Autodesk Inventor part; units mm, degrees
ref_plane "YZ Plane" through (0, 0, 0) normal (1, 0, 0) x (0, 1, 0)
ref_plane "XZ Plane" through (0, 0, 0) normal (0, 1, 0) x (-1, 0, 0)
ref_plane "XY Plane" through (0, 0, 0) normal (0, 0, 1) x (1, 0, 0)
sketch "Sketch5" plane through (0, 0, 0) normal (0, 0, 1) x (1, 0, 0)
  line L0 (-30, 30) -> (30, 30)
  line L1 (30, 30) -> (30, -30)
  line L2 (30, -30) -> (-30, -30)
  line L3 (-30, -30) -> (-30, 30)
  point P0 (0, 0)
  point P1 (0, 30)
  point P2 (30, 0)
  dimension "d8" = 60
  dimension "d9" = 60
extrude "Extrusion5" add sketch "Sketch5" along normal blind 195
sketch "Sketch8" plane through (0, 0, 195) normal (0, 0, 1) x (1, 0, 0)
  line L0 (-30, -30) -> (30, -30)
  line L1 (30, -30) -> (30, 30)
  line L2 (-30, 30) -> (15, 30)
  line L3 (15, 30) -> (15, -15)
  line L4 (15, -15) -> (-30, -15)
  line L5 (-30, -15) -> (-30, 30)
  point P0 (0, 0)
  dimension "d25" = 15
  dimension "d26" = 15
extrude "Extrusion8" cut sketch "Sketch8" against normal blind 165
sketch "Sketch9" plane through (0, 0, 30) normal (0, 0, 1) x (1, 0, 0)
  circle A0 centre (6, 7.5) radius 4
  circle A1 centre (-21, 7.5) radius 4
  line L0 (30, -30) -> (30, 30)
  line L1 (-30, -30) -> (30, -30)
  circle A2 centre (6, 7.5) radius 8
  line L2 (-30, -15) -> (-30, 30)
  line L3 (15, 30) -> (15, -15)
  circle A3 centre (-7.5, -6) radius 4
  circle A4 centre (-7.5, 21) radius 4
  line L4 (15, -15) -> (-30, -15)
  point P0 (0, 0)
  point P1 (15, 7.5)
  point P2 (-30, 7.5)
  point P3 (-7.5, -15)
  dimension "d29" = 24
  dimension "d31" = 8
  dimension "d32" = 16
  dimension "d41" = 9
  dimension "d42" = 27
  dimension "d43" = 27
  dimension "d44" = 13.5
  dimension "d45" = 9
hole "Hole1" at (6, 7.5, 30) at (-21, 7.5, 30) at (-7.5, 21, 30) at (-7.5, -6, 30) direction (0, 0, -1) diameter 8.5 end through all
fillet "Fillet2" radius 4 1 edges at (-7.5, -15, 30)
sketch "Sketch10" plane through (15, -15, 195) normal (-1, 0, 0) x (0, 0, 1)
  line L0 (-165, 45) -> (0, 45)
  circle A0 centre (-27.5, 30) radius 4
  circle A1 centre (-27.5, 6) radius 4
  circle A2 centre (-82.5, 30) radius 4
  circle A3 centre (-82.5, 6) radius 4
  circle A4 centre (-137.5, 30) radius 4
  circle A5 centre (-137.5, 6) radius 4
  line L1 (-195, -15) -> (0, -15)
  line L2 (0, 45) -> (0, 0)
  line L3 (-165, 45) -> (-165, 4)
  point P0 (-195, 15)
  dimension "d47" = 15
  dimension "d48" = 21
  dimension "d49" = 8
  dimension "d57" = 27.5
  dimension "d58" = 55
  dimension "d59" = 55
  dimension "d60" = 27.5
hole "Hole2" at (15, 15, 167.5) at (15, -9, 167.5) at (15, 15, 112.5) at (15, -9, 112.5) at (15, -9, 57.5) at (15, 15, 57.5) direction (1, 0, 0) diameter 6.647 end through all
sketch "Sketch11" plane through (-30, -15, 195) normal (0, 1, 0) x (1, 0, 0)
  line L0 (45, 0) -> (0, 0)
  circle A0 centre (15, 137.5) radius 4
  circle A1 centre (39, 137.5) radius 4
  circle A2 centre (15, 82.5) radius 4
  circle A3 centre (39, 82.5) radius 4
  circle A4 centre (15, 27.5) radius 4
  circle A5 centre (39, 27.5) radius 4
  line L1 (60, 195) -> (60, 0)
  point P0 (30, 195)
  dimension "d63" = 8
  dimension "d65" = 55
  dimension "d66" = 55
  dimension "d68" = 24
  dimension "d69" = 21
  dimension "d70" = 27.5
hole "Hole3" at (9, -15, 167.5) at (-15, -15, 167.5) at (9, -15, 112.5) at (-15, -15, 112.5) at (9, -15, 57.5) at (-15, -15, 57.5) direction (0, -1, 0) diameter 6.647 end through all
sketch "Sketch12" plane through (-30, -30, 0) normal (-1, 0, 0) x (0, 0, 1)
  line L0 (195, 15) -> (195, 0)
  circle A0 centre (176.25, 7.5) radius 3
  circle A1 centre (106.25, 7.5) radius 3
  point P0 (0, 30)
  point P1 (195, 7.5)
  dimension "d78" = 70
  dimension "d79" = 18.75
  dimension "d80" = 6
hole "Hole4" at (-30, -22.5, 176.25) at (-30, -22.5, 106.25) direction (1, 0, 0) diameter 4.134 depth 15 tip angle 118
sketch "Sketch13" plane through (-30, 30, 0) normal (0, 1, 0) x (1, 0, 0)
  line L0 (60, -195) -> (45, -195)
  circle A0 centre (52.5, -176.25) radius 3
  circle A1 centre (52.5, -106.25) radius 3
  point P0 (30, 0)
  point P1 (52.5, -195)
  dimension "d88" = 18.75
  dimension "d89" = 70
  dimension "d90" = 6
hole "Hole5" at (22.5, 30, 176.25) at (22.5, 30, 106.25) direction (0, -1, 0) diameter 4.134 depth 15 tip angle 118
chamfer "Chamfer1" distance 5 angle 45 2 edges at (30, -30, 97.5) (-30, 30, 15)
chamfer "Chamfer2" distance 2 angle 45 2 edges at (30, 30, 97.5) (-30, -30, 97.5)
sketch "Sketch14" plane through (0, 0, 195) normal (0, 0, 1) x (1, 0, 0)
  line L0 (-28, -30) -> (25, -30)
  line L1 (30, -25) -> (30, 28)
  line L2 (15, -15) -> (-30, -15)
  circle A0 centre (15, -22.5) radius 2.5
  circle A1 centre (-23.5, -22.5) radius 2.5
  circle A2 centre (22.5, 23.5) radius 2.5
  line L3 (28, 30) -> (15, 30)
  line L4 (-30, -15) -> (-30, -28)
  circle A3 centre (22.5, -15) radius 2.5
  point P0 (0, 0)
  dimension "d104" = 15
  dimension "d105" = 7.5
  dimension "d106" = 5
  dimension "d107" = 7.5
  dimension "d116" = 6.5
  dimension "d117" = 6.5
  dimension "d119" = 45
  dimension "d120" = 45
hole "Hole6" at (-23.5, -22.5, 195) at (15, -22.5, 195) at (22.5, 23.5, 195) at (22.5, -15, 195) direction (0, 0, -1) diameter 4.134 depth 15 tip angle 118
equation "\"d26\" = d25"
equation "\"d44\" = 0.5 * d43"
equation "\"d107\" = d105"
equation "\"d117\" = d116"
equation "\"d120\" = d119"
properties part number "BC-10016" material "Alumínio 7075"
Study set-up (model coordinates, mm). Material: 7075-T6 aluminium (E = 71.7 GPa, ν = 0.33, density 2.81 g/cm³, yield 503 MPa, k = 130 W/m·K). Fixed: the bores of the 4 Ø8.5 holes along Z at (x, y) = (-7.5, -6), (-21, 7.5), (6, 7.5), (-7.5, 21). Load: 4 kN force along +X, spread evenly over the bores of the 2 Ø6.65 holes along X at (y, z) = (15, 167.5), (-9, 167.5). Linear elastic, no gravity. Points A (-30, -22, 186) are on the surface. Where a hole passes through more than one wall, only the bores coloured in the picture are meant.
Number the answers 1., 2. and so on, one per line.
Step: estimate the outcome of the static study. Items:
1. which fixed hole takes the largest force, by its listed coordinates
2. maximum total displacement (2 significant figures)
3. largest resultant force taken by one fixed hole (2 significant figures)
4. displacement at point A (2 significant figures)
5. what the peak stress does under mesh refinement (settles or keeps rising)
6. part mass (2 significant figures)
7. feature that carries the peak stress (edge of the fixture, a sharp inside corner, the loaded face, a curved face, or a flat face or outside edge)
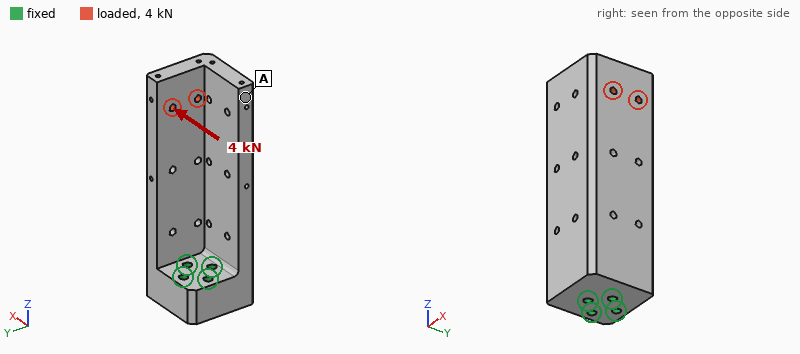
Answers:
1. (6, 7.5)
2. 0.70 mm
3. 8.5 kN
4. 0.40 mm
5. keeps rising
6. 980 g
7. edge of the fixture
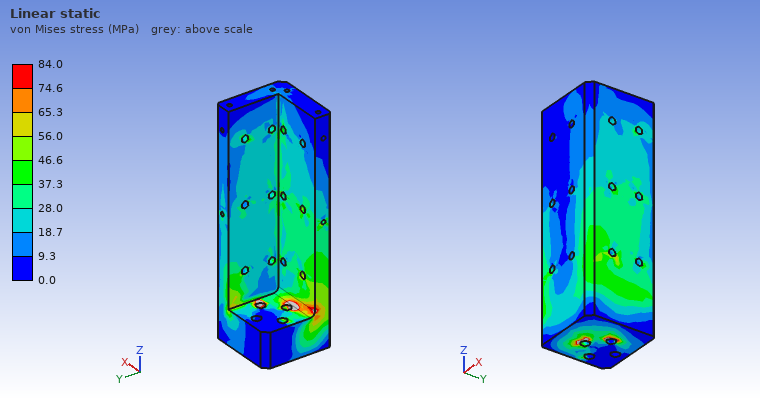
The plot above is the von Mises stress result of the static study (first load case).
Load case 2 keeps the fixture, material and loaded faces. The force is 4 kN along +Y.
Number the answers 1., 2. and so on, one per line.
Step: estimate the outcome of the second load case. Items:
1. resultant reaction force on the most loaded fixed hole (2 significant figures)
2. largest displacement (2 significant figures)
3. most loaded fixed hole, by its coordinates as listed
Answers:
1. 9.1 kN
2. 0.48 mm
3. (-7.5, -6)
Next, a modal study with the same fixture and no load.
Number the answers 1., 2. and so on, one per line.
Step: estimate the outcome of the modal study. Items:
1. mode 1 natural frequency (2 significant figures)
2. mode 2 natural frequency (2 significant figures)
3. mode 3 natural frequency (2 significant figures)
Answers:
1. 790 Hz
2. 1100 Hz
3. 2100 Hz
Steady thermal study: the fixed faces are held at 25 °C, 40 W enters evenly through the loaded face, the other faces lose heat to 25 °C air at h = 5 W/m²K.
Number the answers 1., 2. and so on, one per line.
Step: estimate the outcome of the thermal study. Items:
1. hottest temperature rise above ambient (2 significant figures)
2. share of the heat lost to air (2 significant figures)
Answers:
1. 35 K
2. 11 %
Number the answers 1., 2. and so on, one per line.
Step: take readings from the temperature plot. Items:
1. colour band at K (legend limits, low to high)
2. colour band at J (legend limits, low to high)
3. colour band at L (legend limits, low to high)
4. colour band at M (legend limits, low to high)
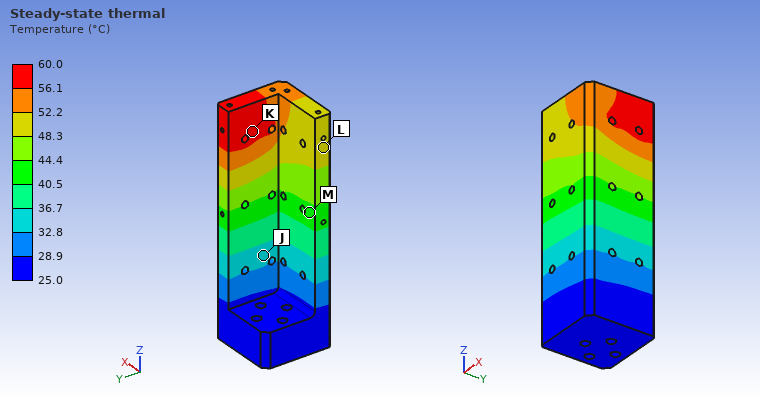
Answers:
1. 56.1 to 60.0 °C
2. 32.8 to 36.7 °C
3. 48.3 to 52.2 °C
4. 40.5 to 44.4 °C
